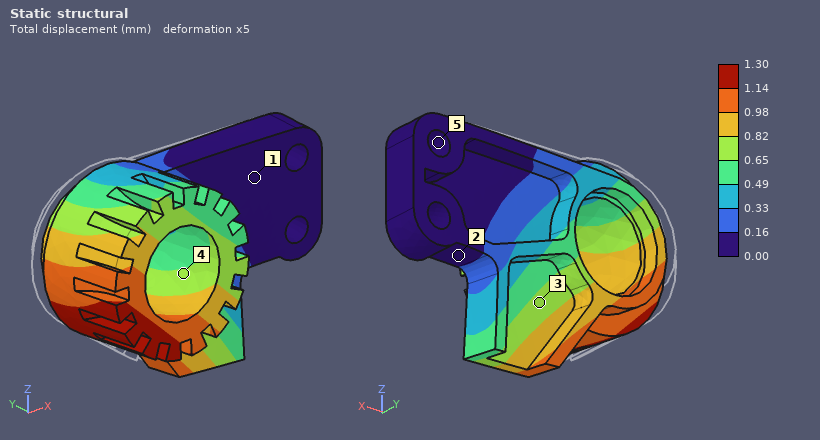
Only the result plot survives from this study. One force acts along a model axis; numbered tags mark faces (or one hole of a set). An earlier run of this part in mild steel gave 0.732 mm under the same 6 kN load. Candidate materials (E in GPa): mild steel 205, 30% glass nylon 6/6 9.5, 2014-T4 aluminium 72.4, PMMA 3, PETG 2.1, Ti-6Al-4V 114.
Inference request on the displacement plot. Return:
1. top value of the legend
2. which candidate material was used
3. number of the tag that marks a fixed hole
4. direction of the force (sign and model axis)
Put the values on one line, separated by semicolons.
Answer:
1.30 mm; Ti-6Al-4V; 5; -Y
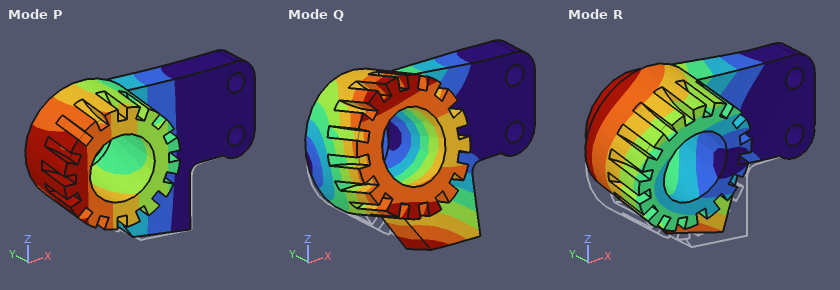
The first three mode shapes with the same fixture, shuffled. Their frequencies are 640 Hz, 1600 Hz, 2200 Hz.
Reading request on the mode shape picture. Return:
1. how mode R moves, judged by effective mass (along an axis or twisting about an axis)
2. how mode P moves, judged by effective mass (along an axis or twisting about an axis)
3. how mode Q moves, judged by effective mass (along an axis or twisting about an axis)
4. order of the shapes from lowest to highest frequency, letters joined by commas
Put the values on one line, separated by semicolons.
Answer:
along Z; along Y; along Z; P, Q, R
